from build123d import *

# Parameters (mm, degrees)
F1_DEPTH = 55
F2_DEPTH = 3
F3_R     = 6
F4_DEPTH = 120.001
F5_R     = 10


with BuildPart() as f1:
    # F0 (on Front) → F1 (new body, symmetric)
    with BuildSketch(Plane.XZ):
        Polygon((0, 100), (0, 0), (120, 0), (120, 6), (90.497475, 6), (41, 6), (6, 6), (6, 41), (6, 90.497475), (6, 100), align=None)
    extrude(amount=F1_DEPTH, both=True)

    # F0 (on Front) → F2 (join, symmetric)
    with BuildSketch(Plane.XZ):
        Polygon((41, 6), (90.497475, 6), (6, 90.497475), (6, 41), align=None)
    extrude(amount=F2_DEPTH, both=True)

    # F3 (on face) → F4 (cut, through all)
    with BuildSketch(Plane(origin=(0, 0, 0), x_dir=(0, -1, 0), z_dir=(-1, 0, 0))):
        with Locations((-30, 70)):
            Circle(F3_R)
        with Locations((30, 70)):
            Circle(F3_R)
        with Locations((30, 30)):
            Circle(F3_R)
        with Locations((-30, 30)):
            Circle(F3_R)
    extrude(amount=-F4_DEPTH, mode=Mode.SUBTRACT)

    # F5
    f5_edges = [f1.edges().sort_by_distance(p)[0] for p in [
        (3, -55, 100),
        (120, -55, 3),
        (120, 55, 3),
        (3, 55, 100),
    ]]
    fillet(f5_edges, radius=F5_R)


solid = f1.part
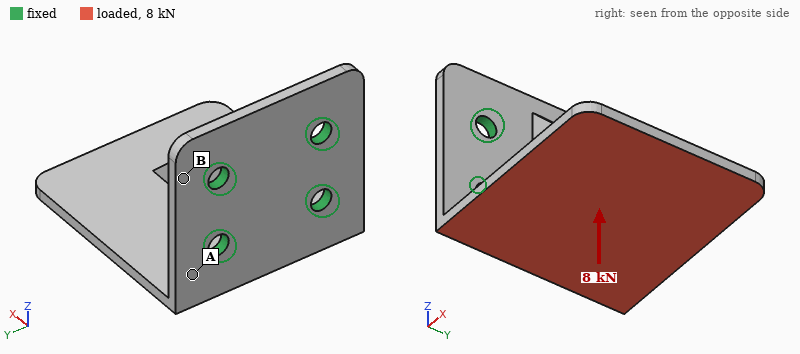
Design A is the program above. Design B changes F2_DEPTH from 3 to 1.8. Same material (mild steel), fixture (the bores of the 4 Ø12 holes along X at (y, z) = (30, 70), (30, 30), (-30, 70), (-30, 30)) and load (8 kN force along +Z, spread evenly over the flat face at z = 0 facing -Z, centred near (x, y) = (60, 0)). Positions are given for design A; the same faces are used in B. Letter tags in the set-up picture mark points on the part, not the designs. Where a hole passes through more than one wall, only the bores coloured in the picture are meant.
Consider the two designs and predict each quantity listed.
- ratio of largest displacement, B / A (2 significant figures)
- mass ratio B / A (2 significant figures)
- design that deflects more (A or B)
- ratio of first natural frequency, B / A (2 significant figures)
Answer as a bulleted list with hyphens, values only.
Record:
- 1.1
- 0.95
- B
- 0.92
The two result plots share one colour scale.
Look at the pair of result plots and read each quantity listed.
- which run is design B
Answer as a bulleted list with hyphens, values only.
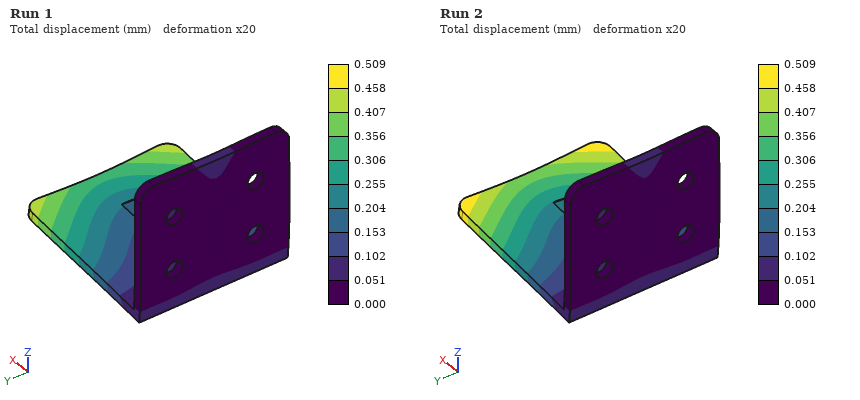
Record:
- Run 2
